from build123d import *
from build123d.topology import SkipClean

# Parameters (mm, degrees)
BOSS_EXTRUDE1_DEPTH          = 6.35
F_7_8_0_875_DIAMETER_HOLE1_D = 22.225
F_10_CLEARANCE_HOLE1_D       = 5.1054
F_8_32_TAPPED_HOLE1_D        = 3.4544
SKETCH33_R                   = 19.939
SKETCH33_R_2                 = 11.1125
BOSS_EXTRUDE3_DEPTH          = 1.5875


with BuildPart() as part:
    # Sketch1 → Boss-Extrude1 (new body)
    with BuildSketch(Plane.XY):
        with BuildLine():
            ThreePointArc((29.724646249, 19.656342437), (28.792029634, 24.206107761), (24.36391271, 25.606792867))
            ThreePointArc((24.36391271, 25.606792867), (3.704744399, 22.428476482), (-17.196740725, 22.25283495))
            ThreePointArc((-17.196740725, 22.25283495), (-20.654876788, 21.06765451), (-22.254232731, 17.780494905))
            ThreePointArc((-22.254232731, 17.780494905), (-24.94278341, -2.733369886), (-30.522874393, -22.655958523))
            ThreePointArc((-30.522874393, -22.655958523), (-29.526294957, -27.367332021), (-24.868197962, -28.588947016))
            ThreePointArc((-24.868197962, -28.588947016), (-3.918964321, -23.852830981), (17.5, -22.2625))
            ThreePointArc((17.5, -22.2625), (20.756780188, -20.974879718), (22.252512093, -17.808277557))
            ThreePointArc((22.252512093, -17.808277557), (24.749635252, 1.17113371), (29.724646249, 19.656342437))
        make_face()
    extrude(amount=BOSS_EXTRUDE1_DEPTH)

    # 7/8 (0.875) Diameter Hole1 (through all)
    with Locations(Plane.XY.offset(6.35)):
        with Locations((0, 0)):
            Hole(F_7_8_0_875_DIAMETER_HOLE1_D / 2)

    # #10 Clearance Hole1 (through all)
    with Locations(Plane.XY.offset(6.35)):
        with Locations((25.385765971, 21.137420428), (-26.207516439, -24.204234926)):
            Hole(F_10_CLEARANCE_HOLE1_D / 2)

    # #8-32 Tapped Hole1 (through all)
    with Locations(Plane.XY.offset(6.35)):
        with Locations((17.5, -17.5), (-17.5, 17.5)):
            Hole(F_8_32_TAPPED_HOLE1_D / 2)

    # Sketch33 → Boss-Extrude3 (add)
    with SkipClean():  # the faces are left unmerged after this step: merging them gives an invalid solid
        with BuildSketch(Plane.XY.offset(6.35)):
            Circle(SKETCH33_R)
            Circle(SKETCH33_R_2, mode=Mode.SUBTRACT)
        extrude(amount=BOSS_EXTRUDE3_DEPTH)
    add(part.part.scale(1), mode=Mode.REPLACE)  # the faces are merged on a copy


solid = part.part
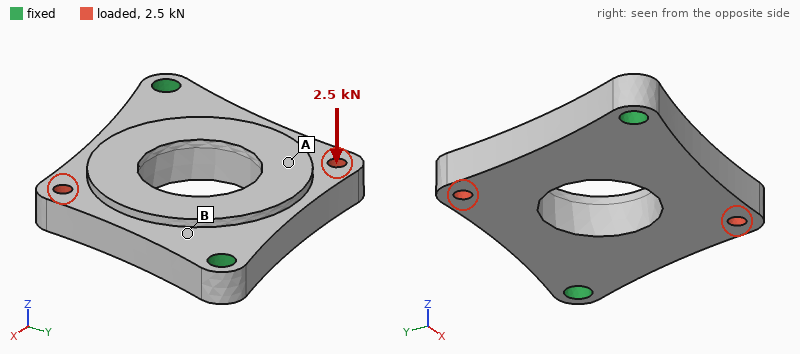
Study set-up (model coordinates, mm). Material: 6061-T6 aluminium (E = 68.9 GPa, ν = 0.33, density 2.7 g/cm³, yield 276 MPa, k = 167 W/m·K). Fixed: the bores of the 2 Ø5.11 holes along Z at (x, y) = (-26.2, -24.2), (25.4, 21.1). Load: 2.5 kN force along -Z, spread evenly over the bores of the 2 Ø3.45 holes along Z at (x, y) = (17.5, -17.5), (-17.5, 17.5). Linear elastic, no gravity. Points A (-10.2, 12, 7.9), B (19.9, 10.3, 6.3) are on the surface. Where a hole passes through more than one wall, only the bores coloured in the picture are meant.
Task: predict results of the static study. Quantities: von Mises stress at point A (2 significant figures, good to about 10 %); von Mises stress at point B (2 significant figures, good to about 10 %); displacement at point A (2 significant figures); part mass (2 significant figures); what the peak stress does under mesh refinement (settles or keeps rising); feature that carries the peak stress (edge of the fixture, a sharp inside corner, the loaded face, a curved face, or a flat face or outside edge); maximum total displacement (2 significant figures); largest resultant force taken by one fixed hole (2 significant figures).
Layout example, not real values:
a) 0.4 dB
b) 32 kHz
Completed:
a) 97 MPa
b) 48 MPa
c) 0.17 mm
d) 37 g
e) keeps rising
f) edge of the fixture
g) 0.28 mm
h) 1.5 kN
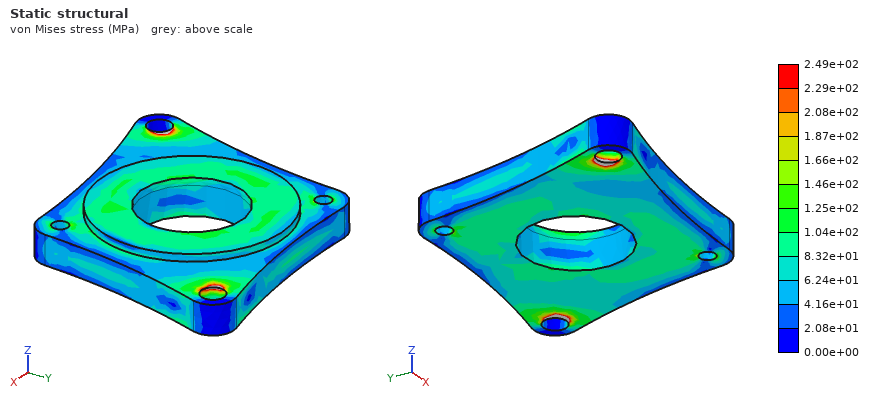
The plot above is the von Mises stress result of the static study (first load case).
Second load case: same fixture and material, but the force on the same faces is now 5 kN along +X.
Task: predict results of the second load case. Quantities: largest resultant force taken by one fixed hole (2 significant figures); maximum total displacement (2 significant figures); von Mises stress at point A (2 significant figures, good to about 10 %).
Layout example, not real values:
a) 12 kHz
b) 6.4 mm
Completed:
a) 2.6 kN
b) 29 µm
c) 16 MPa
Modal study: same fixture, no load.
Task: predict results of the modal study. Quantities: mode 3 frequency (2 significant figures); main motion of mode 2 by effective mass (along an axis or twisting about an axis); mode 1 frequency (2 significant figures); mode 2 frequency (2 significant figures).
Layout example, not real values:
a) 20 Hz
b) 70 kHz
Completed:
a) 13 kHz
b) along Z
c) 4000 Hz
d) 4900 Hz
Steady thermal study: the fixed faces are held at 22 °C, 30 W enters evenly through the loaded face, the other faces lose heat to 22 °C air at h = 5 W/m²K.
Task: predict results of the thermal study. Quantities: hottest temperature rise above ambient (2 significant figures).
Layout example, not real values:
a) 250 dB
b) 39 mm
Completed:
a) 29 K
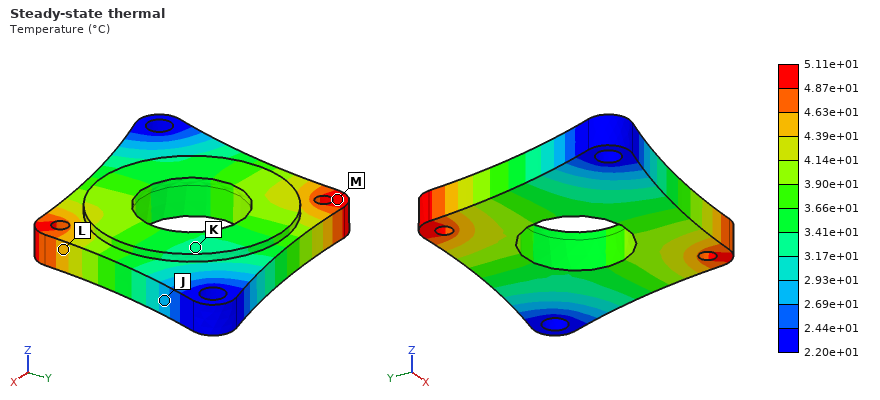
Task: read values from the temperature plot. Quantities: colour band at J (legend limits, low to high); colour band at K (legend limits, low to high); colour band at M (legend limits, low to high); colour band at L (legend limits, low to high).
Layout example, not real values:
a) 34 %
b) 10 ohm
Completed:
a) 2.69e+01 to 2.93e+01 °C
b) 3.17e+01 to 3.41e+01 °C
c) 4.87e+01 to 5.11e+01 °C
d) 4.39e+01 to 4.63e+01 °C
